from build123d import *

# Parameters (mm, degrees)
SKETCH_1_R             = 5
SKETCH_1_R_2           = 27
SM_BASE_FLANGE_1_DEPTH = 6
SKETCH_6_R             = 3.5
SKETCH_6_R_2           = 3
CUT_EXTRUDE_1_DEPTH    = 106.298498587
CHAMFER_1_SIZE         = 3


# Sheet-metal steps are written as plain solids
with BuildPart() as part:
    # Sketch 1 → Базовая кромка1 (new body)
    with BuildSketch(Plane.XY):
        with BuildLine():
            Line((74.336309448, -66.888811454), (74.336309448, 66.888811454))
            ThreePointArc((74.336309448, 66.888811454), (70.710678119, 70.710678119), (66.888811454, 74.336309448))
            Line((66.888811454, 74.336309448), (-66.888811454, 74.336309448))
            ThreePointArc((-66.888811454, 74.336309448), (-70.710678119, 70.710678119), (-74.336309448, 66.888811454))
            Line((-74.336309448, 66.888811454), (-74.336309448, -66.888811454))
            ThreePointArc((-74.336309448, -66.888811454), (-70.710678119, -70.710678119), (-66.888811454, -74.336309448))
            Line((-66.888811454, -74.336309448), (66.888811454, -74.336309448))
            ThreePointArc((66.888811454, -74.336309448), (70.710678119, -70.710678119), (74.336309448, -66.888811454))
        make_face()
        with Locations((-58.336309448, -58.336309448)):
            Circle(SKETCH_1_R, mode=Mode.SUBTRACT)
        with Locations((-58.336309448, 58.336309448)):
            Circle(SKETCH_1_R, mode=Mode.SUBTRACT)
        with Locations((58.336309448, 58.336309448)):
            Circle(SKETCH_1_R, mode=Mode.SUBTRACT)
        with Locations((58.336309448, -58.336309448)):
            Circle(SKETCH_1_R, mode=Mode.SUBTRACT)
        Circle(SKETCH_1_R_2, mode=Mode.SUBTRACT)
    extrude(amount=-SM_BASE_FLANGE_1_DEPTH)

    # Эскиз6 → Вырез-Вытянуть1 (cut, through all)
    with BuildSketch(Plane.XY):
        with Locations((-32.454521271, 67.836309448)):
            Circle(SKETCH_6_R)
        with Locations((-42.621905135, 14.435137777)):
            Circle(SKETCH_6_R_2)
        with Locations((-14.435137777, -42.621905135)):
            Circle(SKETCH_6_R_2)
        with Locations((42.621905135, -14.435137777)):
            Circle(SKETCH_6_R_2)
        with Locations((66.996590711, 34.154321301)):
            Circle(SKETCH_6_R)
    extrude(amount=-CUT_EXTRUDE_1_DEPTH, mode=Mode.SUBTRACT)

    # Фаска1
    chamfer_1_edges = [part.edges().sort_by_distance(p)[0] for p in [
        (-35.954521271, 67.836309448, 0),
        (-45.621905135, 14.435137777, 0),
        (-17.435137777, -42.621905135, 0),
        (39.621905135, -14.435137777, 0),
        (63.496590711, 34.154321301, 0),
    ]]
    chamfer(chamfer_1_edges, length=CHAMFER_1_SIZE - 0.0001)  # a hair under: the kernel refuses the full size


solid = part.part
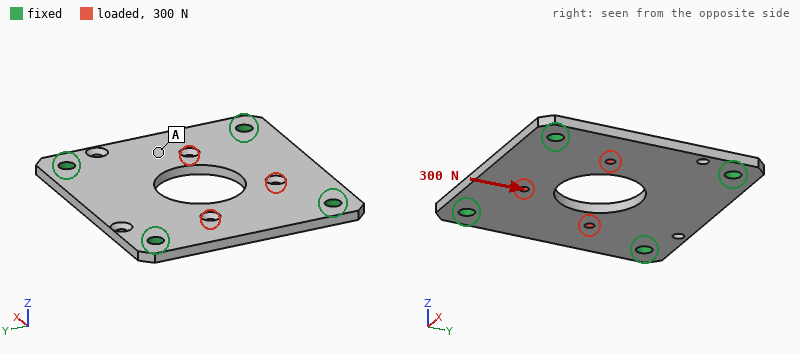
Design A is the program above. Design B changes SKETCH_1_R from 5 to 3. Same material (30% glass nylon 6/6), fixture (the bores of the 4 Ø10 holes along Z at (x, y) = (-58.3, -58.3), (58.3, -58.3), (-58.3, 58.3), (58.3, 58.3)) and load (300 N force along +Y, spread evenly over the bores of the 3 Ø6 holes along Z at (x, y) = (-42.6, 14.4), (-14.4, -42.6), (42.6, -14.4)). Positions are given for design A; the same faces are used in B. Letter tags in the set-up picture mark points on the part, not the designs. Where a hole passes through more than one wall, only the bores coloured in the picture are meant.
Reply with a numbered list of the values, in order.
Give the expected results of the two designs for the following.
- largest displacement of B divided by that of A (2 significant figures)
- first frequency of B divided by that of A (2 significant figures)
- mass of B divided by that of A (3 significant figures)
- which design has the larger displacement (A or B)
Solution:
1. 1.1
2. 0.90
3. 1.01
4. B
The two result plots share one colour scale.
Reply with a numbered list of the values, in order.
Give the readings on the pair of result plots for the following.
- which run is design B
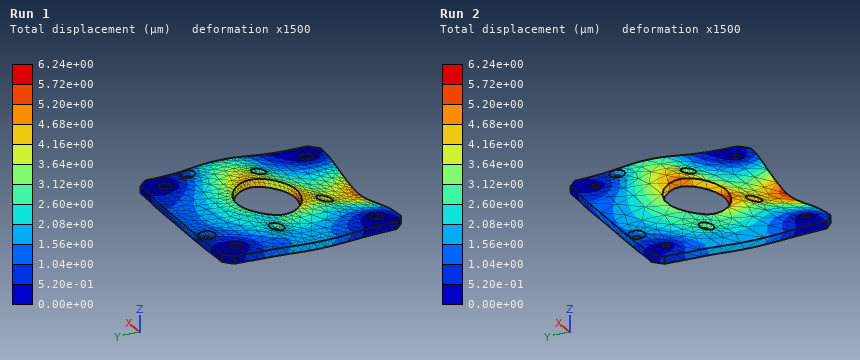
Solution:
1. Run 2
